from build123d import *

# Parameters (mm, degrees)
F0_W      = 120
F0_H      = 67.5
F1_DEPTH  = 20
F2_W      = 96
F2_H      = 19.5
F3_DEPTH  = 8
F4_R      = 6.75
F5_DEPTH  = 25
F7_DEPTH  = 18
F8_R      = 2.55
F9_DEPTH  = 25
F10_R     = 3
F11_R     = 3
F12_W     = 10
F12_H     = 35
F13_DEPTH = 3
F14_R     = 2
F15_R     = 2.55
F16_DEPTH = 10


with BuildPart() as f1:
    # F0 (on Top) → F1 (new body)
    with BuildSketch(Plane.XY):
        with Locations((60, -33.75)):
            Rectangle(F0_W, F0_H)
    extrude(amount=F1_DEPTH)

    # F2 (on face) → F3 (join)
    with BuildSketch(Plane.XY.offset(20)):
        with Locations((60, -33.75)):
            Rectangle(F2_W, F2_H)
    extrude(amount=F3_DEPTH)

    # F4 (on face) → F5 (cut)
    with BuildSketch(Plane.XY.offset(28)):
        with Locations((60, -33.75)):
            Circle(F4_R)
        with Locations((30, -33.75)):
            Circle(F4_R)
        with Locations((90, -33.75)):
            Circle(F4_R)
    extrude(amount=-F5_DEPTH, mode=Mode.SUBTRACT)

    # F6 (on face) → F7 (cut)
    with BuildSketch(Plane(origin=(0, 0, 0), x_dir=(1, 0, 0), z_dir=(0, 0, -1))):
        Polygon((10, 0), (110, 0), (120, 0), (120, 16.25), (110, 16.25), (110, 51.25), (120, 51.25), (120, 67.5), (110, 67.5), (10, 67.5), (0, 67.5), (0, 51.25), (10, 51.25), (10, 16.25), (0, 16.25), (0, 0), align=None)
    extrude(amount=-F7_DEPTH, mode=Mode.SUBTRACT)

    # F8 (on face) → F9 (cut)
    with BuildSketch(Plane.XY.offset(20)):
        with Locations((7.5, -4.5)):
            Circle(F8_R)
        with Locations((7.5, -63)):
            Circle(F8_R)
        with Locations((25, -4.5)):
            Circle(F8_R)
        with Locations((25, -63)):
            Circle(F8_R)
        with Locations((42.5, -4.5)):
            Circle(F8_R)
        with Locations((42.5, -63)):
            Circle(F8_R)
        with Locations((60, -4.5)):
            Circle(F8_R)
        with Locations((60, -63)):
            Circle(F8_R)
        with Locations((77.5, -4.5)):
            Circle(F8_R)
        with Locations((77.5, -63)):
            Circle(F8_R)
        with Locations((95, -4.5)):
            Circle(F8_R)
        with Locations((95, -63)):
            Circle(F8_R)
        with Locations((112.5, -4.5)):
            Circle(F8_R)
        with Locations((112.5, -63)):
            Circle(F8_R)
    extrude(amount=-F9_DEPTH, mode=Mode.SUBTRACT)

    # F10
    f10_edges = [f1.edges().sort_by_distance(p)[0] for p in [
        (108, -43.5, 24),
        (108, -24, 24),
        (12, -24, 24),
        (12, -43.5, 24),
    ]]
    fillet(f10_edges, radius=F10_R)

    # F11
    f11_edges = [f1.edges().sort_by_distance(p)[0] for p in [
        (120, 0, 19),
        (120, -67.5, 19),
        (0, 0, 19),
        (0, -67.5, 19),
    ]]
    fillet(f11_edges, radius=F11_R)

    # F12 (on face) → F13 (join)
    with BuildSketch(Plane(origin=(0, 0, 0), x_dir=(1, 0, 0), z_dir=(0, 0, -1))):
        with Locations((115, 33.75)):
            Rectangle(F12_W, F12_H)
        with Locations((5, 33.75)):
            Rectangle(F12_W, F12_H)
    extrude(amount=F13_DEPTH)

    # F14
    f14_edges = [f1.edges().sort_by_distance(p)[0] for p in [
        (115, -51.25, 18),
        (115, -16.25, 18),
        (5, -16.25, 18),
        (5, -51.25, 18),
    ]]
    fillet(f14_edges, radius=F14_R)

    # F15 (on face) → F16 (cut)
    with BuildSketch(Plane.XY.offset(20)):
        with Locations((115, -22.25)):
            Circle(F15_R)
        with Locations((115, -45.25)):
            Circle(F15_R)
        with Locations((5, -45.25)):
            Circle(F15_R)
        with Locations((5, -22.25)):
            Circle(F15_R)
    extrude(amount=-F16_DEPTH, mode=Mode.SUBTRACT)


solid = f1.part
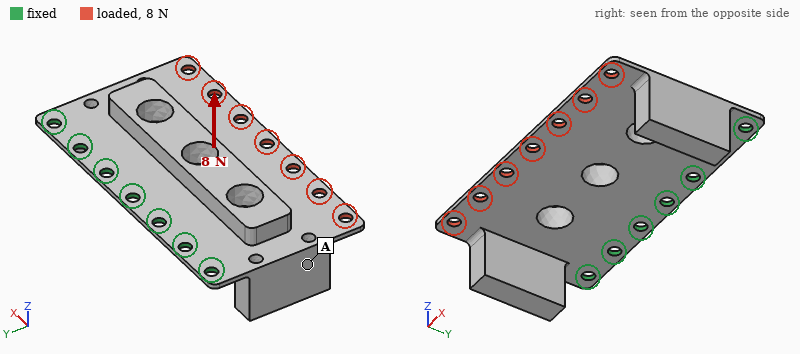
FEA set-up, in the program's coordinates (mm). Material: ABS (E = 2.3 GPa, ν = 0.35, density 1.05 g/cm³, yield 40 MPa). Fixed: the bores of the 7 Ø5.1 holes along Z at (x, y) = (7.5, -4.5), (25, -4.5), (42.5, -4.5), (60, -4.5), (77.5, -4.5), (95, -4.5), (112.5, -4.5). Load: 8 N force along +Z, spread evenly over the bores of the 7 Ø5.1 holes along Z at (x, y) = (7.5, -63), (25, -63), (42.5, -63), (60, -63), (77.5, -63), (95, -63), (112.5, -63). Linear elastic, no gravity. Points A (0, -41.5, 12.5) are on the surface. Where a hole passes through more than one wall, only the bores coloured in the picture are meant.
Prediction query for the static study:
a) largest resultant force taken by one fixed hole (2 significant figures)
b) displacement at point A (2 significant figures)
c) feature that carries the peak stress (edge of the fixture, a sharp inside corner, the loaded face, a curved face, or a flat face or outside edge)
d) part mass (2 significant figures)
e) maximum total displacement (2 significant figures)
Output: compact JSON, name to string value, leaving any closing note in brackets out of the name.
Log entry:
{"largest resultant force taken by one fixed hole": "3.6 N", "displacement at point A": "0.84 mm", "feature that carries the peak stress": "a curved face", "part mass": "42 g", "maximum total displacement": "1.7 mm"}
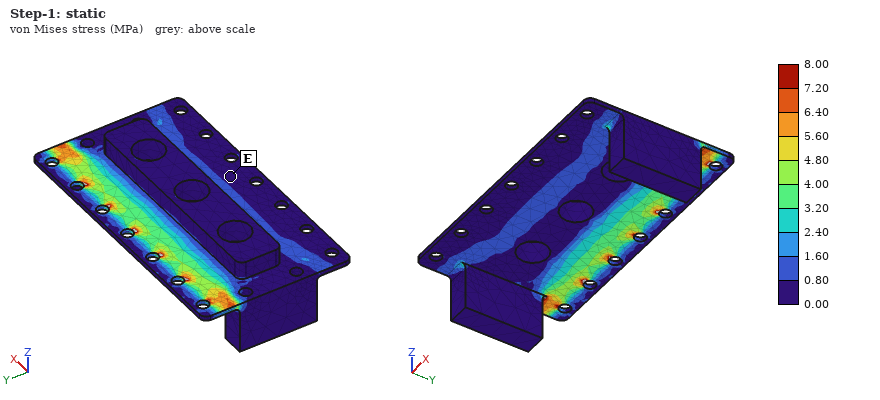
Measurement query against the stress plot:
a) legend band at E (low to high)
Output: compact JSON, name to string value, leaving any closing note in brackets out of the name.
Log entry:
{"legend band at E": "0.00 to 0.80 MPa"}
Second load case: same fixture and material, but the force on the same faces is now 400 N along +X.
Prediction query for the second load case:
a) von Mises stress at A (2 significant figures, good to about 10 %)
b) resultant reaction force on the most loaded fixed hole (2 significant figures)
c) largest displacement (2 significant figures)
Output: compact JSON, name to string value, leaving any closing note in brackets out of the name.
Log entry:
{"von Mises stress at A": "0.74 MPa", "resultant reaction force on the most loaded fixed hole": "170 N", "largest displacement": "0.56 mm"}
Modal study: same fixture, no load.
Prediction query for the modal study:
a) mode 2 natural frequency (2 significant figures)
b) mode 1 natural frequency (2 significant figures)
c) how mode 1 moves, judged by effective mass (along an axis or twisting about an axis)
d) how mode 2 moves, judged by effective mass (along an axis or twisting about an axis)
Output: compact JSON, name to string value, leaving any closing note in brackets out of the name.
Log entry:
{"mode 2 natural frequency": "300 Hz", "mode 1 natural frequency": "110 Hz", "how mode 1 moves, judged by effective mass": "along Z", "how mode 2 moves, judged by effective mass": "twisting about Y"}
